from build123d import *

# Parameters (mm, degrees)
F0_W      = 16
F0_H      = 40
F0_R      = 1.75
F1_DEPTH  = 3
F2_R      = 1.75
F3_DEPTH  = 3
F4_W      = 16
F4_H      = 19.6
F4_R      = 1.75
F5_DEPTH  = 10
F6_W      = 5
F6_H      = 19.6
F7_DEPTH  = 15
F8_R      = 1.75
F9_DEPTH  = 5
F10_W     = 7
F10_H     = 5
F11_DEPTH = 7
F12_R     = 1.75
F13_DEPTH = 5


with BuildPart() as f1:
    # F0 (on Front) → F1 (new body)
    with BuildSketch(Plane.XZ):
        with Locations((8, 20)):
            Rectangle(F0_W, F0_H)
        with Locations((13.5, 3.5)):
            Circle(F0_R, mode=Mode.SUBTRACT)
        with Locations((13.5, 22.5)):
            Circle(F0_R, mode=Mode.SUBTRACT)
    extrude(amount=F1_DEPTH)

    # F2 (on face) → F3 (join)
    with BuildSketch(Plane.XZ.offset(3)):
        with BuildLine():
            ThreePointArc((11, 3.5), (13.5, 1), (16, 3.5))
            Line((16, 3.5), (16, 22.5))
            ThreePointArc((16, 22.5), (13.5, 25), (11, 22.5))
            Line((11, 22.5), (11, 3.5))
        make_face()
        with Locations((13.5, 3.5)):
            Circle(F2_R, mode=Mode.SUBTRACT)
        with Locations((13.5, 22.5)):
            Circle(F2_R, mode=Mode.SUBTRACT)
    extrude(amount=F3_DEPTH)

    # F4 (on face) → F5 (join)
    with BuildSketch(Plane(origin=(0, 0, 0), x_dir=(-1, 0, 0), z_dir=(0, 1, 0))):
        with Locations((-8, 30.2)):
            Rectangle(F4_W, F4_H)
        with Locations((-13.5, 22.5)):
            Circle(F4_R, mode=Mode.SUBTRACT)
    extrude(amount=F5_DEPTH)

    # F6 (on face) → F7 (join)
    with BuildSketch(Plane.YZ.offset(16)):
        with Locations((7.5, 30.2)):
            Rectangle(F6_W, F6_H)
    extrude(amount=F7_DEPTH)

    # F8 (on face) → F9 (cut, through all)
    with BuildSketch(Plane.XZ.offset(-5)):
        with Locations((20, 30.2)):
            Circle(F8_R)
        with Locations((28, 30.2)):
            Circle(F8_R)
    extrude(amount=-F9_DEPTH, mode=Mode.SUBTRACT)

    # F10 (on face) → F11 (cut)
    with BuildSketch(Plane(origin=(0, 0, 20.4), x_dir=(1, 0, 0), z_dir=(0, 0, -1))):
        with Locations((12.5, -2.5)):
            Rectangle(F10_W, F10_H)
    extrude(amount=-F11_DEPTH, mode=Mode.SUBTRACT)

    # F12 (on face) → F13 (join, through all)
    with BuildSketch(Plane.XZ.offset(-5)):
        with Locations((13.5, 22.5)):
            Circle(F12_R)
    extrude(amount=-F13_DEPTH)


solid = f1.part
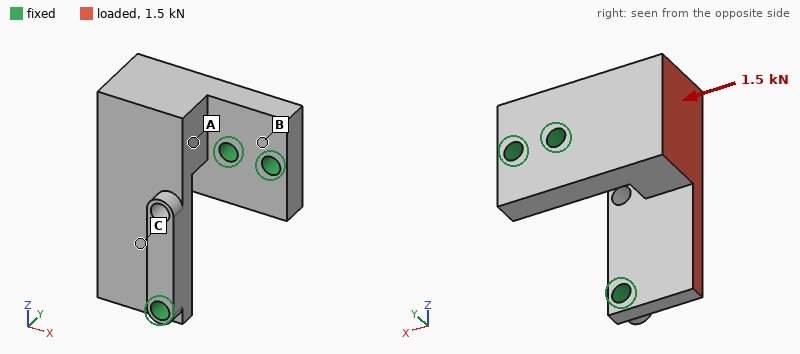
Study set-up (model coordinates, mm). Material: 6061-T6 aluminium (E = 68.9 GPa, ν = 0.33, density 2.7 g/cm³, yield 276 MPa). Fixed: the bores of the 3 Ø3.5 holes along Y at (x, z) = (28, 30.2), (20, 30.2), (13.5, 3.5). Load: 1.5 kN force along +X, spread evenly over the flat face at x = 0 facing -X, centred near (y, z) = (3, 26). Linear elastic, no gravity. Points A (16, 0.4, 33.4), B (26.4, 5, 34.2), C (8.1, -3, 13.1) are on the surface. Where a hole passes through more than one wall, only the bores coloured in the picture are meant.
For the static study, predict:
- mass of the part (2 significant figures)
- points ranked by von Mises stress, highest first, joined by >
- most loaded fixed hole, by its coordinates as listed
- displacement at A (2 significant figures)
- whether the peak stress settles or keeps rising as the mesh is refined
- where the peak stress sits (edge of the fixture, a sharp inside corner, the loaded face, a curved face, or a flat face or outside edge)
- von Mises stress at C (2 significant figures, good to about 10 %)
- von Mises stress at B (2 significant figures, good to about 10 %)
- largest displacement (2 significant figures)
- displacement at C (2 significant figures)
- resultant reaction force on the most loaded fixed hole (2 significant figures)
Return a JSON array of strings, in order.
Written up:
["17 g", "C > B > A", "(20, 30.2)", "13 µm", "keeps rising", "edge of the fixture", "23 MPa", "14 MPa", "34 µm", "10 µm", "990 N"]
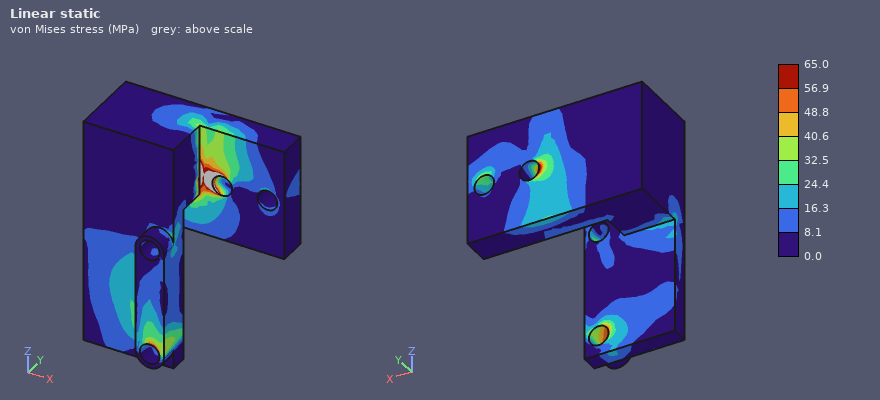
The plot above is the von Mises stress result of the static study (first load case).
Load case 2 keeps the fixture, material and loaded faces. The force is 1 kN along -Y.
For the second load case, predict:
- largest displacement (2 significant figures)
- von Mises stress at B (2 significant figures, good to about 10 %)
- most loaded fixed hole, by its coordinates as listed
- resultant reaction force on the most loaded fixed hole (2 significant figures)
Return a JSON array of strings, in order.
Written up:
["0.10 mm", "25 MPa", "(20, 30.2)", "1.5 kN"]
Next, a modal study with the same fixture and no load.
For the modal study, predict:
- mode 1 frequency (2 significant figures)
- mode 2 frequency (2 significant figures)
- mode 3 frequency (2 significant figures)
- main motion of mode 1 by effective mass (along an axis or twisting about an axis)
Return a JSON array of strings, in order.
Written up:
["7200 Hz", "16 kHz", "21 kHz", "along Y"]
